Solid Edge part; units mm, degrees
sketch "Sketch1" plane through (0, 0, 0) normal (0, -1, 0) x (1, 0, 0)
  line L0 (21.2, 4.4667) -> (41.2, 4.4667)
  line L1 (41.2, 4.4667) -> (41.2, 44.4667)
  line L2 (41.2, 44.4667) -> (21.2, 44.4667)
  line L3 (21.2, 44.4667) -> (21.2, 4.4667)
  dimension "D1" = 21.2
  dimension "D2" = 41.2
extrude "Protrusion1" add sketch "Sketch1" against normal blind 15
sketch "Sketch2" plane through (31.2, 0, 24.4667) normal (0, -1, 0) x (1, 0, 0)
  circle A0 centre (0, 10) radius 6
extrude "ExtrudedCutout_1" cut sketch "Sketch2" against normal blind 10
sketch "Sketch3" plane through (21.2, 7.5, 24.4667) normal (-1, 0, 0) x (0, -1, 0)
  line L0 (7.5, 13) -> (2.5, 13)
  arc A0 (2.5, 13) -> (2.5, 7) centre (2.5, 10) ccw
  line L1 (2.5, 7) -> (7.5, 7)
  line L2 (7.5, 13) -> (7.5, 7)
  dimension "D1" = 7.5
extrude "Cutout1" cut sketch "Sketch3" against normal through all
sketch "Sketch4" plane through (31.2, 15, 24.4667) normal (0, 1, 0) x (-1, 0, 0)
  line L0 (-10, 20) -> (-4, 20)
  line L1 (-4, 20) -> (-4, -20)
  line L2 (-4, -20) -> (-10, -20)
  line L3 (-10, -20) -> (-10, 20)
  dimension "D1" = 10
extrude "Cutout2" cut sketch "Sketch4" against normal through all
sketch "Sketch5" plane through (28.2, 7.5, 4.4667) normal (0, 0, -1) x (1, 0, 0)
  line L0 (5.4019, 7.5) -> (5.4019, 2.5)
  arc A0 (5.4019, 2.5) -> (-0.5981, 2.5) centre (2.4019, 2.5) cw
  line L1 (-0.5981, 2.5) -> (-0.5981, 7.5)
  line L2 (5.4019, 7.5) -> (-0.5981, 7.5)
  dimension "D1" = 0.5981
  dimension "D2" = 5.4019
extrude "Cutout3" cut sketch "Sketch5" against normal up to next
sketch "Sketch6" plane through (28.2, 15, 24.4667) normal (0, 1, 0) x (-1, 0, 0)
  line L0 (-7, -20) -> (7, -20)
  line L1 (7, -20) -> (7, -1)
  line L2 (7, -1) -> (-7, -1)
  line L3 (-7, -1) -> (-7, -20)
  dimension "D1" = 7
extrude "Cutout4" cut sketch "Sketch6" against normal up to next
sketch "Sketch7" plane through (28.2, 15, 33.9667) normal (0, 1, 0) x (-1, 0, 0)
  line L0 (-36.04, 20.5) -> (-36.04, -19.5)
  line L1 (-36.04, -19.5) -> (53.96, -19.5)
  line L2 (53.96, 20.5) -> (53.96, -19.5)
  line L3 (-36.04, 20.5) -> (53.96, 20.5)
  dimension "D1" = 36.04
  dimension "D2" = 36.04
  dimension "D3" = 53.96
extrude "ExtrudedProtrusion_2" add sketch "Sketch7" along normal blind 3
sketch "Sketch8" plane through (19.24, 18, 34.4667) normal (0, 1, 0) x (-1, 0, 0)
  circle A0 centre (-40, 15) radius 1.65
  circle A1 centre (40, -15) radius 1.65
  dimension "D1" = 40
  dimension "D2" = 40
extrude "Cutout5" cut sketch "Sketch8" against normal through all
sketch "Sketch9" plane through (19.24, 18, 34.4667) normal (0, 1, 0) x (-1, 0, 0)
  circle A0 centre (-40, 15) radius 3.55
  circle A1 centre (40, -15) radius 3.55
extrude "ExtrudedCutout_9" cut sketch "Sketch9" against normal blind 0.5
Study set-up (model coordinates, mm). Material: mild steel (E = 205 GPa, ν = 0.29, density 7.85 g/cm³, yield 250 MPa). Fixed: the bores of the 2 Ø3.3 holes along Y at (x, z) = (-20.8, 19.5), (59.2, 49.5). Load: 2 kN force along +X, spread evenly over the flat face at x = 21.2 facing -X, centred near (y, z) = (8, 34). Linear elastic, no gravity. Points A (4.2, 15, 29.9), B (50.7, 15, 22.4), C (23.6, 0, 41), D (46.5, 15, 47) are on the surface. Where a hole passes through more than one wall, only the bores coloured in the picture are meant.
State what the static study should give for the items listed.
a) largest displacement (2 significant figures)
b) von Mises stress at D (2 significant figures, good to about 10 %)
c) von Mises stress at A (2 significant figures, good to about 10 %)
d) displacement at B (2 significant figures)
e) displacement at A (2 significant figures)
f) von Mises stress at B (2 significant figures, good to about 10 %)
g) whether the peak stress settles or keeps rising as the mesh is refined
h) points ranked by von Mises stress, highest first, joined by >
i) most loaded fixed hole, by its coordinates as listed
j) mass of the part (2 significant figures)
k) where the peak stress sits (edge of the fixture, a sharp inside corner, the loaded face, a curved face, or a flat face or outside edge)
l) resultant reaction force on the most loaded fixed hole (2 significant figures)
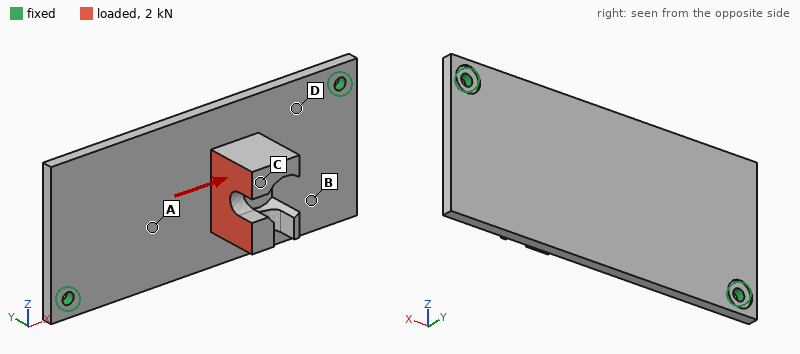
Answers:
0.17 mm
98 MPa
68 MPa
0.099 mm
0.070 mm
38 MPa
keeps rising
D > A > B > C
(59.2, 49.5)
110 g
edge of the fixture
1.2 kN
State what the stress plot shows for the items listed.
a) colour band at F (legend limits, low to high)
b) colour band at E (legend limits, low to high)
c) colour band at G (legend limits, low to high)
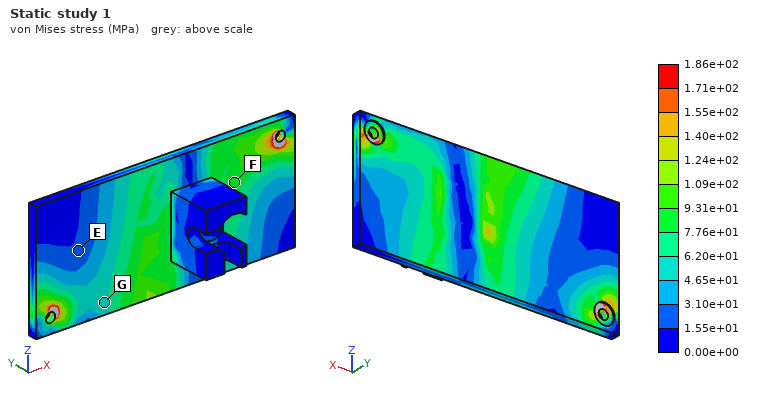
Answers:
7.76e+01 to 9.31e+01 MPa
1.55e+01 to 3.10e+01 MPa
4.65e+01 to 6.20e+01 MPa
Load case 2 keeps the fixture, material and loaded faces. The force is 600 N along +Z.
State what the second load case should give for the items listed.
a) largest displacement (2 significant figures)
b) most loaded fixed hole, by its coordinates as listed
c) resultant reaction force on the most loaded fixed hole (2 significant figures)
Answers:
0.11 mm
(59.2, 49.5)
330 N
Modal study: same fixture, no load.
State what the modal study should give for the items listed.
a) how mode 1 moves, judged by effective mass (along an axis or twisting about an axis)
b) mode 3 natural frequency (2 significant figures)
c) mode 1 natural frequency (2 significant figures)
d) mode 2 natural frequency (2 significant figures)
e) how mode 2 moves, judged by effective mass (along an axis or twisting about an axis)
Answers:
along Y
3300 Hz
1300 Hz
1400 Hz
along Y
